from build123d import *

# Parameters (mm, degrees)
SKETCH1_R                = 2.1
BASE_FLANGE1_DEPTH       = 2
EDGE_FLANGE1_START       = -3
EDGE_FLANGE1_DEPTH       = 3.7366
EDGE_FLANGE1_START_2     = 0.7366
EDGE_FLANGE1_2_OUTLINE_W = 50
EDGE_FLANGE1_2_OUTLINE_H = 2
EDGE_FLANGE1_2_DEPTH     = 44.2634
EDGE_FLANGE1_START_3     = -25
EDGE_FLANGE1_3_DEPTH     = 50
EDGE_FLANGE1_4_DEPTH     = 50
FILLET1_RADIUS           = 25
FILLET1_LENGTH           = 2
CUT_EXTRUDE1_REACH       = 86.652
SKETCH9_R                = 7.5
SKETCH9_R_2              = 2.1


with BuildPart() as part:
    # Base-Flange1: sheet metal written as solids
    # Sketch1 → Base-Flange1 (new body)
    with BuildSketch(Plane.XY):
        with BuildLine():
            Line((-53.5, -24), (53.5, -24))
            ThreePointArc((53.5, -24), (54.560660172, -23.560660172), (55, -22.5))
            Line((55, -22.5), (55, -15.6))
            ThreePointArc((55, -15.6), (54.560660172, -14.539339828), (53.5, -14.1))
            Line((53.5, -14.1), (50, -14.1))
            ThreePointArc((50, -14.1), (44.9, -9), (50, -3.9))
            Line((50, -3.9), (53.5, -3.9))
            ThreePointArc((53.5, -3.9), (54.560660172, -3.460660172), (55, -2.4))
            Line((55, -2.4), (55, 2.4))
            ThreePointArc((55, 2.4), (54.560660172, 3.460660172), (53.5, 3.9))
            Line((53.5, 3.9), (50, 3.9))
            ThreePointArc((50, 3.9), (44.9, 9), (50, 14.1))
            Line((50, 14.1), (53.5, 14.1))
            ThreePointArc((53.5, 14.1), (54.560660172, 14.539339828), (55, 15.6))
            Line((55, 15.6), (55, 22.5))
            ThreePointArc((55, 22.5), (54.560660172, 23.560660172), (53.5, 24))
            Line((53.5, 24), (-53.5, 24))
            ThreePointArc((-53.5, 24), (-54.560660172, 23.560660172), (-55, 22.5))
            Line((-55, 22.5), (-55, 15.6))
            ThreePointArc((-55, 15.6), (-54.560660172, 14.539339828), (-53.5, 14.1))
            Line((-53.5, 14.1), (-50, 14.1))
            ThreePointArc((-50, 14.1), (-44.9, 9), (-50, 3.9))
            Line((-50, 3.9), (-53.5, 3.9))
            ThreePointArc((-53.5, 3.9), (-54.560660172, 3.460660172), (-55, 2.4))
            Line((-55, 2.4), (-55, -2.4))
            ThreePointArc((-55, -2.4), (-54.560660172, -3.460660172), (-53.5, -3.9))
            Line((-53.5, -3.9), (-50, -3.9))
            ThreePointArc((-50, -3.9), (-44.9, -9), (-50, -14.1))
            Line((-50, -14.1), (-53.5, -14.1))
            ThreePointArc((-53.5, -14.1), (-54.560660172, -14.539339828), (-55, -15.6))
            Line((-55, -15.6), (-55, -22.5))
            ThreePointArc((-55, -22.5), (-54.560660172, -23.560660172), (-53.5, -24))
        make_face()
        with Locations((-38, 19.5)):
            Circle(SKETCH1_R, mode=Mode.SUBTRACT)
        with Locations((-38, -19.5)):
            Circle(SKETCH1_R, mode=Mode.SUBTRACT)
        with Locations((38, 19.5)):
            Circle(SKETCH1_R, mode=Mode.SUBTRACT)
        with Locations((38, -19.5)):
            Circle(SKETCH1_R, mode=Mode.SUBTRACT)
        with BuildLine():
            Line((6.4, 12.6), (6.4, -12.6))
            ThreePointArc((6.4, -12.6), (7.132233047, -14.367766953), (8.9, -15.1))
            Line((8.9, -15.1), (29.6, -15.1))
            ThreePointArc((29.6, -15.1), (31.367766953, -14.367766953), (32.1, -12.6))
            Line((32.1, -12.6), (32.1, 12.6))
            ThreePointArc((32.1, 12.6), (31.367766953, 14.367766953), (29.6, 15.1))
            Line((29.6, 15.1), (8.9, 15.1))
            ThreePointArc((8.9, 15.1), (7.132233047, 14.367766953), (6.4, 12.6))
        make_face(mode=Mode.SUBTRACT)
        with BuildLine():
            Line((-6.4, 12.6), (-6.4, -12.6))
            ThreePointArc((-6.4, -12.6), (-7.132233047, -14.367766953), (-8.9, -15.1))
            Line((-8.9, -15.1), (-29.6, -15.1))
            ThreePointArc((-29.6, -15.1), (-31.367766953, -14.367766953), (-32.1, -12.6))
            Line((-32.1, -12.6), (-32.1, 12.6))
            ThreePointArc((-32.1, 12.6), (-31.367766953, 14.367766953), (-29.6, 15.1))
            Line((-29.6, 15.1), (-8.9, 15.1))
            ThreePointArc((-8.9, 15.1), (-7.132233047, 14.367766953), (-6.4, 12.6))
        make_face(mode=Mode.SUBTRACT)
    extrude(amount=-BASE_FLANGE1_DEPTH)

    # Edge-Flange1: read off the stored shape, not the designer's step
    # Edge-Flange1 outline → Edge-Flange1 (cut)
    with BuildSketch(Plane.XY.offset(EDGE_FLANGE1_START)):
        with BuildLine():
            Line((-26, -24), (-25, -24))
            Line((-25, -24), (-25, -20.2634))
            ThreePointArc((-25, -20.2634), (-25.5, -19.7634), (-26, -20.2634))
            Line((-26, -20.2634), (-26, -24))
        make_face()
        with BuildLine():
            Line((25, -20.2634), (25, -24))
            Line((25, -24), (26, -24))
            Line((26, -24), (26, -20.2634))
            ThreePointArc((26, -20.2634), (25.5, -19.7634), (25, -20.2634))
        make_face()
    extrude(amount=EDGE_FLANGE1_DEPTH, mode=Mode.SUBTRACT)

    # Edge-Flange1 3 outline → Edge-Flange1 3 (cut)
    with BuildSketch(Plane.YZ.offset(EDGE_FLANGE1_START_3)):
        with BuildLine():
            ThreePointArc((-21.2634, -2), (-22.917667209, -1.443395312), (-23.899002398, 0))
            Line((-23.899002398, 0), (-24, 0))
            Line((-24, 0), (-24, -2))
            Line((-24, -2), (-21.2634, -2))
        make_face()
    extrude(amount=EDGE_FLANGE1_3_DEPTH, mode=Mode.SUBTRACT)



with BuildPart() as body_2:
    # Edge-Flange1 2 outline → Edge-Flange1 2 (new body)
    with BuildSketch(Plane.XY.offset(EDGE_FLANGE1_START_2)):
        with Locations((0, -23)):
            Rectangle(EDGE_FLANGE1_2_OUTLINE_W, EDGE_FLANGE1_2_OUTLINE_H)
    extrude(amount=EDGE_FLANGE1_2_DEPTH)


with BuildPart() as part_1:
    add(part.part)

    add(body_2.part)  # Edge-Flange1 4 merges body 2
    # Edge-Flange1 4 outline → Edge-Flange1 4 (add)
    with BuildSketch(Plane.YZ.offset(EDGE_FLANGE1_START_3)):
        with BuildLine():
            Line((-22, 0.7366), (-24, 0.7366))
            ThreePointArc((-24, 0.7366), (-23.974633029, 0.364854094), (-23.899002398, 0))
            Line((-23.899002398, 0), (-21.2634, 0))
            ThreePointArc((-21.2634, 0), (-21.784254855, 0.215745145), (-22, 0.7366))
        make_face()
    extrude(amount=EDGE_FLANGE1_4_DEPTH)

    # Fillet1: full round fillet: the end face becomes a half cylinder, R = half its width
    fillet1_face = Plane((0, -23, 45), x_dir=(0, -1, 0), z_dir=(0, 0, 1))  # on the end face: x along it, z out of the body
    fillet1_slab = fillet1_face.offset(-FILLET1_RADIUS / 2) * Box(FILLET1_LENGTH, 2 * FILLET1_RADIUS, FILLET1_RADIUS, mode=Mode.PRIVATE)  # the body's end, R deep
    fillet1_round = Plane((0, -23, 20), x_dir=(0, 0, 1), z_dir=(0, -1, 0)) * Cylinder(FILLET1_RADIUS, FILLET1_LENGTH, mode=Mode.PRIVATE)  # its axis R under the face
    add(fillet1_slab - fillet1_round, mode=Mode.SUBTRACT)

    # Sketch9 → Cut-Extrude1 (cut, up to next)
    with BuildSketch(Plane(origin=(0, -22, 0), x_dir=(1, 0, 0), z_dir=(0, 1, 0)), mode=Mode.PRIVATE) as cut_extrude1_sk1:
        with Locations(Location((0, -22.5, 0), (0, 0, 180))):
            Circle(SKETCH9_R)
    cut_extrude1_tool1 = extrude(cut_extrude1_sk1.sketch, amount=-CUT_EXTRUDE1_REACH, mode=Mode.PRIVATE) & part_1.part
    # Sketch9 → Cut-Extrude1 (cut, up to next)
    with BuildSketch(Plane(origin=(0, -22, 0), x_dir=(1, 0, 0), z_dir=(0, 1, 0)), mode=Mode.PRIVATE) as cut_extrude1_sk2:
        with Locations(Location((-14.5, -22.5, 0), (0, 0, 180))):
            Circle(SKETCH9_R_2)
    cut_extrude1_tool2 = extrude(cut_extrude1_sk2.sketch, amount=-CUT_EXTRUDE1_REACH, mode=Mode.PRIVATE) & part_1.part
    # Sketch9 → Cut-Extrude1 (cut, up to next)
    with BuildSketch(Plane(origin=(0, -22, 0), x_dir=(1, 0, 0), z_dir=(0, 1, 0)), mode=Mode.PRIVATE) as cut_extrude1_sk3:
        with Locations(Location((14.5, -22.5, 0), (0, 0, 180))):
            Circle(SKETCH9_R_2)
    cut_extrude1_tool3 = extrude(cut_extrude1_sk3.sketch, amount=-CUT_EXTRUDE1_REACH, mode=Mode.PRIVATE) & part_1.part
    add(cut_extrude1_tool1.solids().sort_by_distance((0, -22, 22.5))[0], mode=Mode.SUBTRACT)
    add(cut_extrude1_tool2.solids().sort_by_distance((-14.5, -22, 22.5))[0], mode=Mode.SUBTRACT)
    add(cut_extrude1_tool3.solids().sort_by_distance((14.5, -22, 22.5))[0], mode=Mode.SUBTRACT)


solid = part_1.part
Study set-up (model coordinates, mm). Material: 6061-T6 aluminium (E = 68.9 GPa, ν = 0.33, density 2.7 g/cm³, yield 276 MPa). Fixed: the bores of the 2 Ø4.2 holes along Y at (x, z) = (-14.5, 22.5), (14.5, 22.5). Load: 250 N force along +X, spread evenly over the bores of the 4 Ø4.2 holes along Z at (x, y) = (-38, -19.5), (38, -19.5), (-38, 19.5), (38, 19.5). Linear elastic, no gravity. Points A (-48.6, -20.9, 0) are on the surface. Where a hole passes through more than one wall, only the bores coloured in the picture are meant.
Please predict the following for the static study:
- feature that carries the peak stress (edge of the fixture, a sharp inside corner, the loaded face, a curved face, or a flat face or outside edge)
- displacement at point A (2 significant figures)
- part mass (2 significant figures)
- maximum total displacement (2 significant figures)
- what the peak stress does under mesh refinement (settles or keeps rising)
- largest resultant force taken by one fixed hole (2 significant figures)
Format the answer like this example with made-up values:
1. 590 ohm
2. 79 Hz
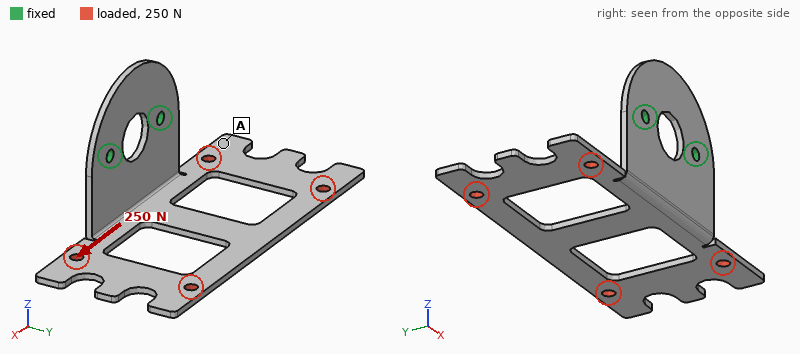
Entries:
1. edge of the fixture
2. 0.82 mm
3. 27 g
4. 1.3 mm
5. keeps rising
6. 260 N
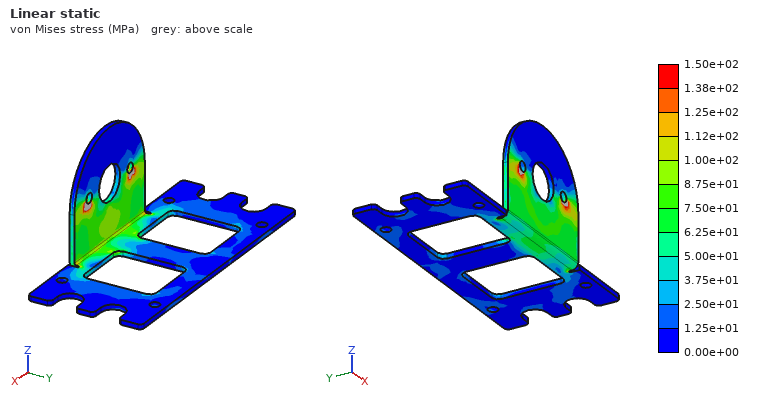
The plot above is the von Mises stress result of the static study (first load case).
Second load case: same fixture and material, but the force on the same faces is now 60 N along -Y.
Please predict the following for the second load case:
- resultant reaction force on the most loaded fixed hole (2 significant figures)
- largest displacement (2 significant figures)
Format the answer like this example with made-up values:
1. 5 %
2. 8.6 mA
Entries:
1. 30 N
2. 0.39 mm
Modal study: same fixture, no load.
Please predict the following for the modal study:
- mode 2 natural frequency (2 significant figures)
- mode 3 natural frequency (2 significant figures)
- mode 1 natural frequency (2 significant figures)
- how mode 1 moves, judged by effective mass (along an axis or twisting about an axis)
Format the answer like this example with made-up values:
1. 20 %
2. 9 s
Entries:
1. 410 Hz
2. 550 Hz
3. 280 Hz
4. along Z
